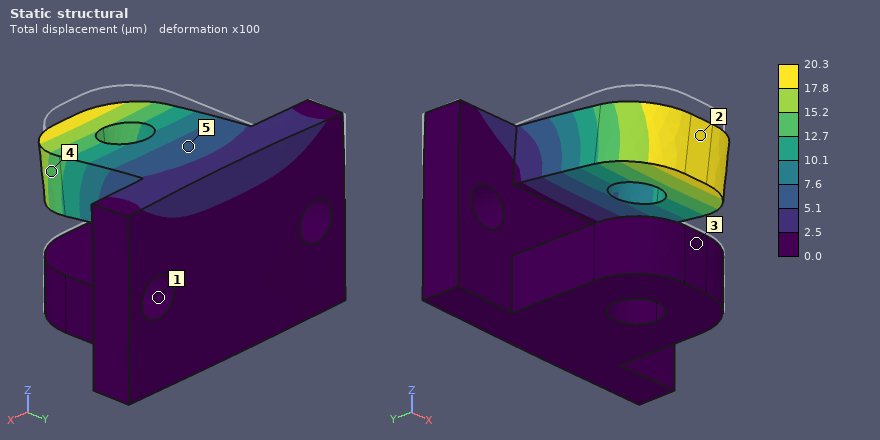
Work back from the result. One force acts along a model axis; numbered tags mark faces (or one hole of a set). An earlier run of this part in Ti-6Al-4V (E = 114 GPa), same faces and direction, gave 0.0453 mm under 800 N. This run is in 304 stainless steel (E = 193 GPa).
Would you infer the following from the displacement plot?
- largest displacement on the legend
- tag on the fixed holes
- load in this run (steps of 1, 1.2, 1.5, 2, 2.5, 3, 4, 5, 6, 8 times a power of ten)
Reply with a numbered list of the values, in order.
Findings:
1. 20.3 µm
2. 1
3. 600 N
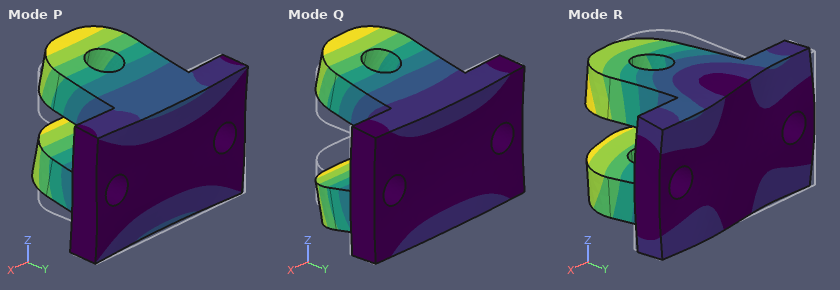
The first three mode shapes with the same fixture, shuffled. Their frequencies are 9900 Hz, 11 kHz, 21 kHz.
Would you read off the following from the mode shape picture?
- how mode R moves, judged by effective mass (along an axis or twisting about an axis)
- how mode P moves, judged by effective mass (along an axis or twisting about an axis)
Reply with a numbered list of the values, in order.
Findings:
1. along X
2. along Z
